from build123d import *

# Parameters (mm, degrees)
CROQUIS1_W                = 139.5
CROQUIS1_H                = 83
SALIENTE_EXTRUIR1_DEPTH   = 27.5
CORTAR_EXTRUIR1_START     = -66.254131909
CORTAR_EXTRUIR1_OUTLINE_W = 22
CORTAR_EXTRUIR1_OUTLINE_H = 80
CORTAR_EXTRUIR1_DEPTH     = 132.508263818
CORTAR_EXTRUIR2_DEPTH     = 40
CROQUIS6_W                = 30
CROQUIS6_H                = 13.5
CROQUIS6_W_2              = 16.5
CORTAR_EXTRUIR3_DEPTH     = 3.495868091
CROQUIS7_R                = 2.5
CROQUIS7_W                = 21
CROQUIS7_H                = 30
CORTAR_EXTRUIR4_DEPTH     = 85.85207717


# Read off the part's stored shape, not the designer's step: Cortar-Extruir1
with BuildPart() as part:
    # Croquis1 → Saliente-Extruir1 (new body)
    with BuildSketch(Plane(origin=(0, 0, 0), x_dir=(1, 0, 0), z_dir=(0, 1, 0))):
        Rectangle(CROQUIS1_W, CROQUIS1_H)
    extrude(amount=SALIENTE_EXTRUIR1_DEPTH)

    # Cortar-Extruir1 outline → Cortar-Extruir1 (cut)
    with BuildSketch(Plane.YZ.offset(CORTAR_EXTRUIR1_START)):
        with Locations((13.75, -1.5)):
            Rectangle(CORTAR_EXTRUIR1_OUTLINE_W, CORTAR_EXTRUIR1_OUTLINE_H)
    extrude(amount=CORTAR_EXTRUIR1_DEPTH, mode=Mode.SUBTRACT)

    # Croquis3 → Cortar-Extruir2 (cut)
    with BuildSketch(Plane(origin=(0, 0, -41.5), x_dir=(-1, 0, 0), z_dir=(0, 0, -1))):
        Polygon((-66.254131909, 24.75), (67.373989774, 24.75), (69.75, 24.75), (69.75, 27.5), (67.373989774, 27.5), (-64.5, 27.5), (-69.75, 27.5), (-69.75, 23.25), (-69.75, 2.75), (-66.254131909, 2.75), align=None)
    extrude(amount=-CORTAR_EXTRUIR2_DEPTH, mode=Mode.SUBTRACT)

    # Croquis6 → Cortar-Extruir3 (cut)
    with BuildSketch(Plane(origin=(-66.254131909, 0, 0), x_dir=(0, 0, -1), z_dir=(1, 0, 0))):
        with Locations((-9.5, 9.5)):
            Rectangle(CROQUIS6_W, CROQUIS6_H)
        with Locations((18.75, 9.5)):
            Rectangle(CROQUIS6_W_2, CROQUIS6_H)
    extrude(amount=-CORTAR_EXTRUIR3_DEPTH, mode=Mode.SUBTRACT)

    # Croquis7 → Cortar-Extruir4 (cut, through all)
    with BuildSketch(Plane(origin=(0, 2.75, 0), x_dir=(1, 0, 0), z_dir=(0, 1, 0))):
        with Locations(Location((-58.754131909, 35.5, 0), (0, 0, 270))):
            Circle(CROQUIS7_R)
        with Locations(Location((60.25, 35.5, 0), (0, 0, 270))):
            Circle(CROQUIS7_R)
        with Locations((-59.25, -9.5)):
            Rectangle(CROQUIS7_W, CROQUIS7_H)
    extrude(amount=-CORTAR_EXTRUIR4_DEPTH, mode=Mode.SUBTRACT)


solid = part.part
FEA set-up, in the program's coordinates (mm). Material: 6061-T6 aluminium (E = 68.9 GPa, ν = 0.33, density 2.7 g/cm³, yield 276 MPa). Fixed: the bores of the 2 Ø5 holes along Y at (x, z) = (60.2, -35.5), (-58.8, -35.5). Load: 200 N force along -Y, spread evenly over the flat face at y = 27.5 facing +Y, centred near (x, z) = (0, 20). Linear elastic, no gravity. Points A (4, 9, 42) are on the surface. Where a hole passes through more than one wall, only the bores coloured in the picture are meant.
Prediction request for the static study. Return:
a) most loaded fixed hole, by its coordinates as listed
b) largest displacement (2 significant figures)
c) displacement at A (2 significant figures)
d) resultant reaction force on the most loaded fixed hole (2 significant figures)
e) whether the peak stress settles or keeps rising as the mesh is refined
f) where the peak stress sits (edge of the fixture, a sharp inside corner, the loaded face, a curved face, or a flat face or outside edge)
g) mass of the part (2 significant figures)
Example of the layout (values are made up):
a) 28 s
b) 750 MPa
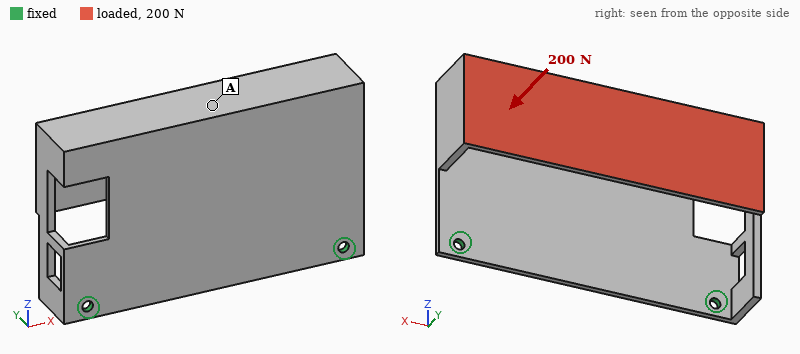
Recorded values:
a) (-58.8, -35.5)
b) 1.1 mm
c) 0.93 mm
d) 110 N
e) keeps rising
f) edge of the fixture
g) 170 g
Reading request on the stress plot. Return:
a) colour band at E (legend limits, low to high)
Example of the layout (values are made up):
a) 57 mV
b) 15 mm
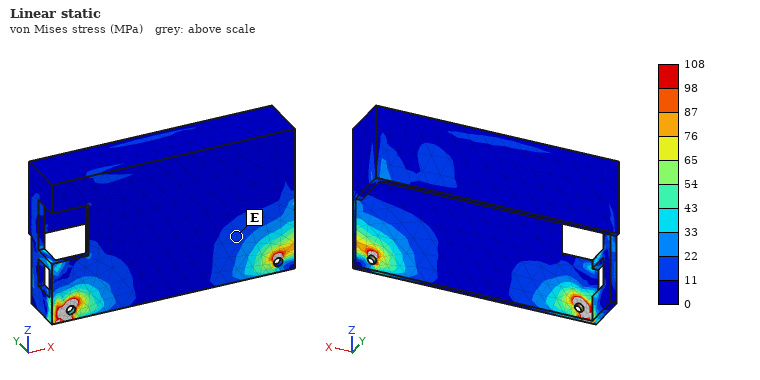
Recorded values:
a) 11 to 22 MPa
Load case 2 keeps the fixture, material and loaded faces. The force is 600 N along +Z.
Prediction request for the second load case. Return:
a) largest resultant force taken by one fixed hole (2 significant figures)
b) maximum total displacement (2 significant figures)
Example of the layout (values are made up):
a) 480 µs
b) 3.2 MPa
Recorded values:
a) 330 N
b) 1.8 mm
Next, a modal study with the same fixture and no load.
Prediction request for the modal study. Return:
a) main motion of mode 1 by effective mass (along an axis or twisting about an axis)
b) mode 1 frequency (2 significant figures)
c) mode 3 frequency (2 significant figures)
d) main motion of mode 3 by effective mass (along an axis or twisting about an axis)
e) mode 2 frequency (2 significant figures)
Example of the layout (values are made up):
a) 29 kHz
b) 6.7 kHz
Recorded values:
a) along Y
b) 210 Hz
c) 1100 Hz
d) along Y
e) 500 Hz
